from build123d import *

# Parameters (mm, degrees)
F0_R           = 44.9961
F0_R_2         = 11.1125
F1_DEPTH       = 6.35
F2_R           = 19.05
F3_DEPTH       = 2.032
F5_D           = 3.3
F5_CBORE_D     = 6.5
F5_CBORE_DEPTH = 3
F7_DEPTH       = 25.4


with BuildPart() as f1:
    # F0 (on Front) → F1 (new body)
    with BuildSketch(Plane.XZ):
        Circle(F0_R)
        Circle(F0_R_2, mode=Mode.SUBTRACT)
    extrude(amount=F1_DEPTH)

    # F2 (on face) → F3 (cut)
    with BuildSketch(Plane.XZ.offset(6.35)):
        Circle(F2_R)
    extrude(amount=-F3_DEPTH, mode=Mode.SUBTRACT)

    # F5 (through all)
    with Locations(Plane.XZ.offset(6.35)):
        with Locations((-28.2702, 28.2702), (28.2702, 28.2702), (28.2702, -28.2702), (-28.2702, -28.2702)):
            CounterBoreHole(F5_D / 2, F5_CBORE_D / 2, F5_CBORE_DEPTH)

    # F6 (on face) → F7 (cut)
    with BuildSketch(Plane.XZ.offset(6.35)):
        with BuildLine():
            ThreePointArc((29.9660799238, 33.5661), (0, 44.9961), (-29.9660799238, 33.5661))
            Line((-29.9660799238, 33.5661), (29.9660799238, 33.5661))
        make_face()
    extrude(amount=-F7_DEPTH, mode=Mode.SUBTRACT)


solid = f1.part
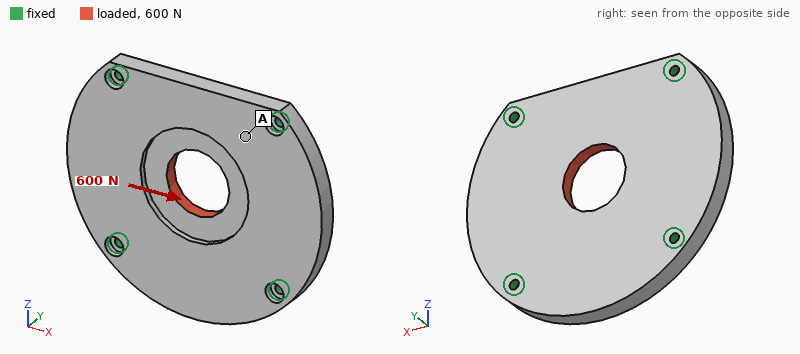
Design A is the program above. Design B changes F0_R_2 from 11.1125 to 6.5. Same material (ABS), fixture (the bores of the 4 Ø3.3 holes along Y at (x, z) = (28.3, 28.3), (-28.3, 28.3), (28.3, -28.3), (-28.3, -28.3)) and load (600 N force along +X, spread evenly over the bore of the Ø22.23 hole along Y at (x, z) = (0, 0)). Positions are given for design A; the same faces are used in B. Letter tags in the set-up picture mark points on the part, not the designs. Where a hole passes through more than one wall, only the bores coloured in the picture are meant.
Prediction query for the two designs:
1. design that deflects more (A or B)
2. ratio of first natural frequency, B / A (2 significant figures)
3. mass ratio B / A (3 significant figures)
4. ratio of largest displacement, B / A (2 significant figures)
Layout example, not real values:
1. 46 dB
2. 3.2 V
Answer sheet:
1. B
2. 0.96
3. 1.03
4. 1.2
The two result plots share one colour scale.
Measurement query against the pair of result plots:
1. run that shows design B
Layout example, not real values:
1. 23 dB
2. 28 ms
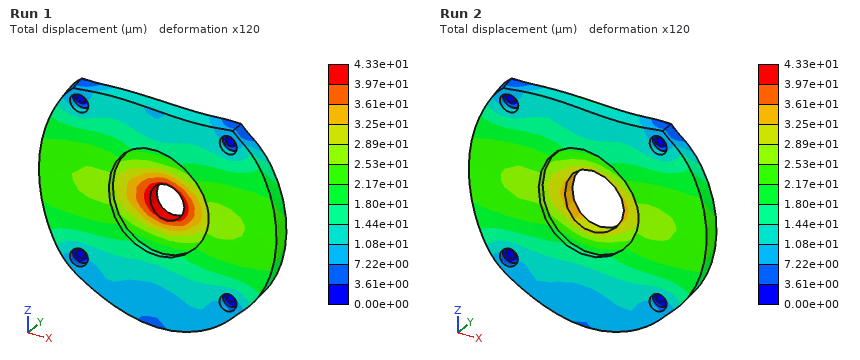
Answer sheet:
1. Run 1
